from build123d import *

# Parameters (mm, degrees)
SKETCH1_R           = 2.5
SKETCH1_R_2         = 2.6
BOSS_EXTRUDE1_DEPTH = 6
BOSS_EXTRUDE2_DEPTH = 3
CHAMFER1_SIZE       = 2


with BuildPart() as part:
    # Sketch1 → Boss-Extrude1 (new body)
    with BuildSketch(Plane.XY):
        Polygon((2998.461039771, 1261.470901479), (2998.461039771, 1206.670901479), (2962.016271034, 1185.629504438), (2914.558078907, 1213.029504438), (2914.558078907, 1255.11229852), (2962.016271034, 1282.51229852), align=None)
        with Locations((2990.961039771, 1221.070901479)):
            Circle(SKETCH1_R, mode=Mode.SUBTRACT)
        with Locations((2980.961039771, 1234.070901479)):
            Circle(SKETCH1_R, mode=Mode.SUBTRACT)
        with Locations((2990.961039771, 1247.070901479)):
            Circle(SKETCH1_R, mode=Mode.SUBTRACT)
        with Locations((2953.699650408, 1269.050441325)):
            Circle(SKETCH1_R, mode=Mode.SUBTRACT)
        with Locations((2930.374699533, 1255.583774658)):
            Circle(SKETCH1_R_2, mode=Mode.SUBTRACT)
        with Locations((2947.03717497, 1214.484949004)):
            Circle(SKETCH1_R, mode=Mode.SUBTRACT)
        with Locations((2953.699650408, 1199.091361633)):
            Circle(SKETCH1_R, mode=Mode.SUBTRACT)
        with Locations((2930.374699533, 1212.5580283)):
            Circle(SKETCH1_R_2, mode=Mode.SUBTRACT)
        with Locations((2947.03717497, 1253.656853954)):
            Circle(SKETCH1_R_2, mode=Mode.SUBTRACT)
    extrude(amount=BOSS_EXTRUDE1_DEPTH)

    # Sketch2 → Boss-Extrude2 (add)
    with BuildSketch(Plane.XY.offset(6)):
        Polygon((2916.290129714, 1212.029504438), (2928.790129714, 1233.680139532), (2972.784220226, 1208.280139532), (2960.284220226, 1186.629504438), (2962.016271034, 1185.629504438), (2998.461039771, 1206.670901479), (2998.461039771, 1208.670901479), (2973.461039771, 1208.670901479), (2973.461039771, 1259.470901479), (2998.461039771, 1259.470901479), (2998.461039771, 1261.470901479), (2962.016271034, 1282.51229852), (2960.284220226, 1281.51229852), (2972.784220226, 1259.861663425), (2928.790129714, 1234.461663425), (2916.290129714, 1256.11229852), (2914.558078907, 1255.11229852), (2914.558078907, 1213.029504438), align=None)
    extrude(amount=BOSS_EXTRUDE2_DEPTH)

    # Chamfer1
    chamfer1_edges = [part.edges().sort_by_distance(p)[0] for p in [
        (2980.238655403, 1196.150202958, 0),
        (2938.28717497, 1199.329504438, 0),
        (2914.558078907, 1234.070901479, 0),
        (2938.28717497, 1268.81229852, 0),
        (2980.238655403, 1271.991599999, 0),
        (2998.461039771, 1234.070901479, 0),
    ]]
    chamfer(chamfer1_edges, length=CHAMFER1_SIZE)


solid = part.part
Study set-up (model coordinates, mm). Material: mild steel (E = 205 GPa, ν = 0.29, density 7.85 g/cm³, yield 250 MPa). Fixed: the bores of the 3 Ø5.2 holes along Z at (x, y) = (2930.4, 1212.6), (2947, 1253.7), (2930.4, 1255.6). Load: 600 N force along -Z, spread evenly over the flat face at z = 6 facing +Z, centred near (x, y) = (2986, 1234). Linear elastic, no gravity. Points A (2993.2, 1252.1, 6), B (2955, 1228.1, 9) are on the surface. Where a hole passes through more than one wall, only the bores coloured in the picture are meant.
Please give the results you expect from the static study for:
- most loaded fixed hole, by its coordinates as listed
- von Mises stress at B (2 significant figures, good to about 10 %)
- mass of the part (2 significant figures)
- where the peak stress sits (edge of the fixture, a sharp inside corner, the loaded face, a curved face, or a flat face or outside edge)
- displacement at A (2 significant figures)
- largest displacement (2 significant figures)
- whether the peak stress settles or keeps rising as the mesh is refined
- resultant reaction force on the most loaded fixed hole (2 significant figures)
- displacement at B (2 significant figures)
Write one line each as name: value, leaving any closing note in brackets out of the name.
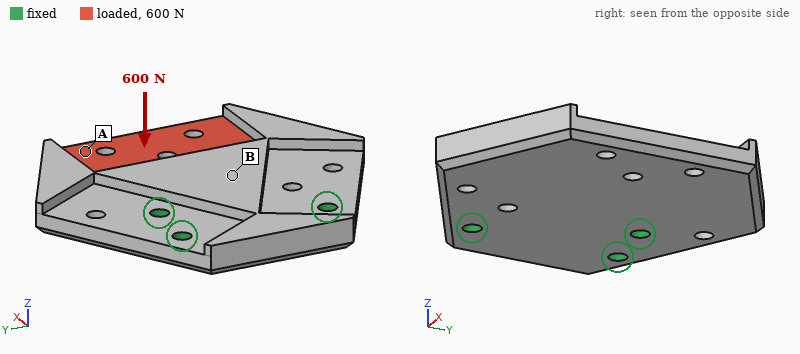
most loaded fixed hole, by its coordinates as listed: (2947, 1253.7)
von Mises stress at B: 28 MPa
mass of the part: 330 g
where the peak stress sits: edge of the fixture
displacement at A: 51 µm
largest displacement: 77 µm
whether the peak stress settles or keeps rising as the mesh is refined: keeps rising
resultant reaction force on the most loaded fixed hole: 1.0 kN
displacement at B: 15 µm
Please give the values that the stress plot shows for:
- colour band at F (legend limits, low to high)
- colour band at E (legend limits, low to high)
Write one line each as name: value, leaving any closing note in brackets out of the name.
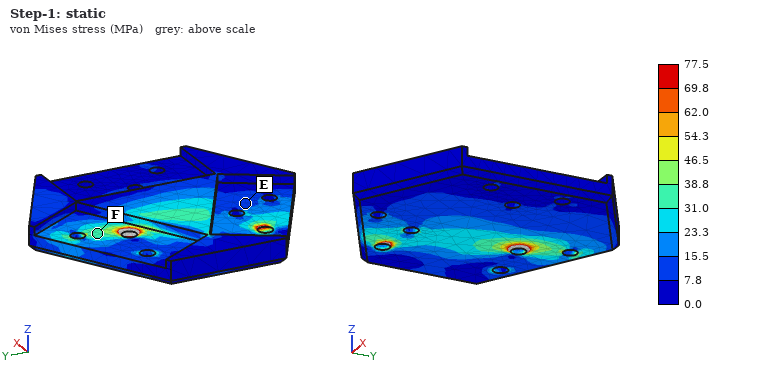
colour band at F: 31.0 to 38.8 MPa
colour band at E: 7.8 to 15.5 MPa
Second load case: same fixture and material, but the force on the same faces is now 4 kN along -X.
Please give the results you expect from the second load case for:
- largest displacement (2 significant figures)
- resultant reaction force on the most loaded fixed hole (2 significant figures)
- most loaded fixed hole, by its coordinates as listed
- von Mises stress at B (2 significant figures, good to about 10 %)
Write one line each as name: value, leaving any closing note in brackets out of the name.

largest displacement: 41 µm
resultant reaction force on the most loaded fixed hole: 1.8 kN
most loaded fixed hole, by its coordinates as listed: (2930.4, 1212.6)
von Mises stress at B: 19 MPa
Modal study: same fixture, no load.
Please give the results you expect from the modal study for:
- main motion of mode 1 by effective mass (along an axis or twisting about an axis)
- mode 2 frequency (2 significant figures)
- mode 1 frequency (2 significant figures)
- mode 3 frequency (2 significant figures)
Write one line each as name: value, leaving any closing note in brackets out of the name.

main motion of mode 1 by effective mass: along Z
mode 2 frequency: 3200 Hz
mode 1 frequency: 1600 Hz
mode 3 frequency: 6000 Hz
